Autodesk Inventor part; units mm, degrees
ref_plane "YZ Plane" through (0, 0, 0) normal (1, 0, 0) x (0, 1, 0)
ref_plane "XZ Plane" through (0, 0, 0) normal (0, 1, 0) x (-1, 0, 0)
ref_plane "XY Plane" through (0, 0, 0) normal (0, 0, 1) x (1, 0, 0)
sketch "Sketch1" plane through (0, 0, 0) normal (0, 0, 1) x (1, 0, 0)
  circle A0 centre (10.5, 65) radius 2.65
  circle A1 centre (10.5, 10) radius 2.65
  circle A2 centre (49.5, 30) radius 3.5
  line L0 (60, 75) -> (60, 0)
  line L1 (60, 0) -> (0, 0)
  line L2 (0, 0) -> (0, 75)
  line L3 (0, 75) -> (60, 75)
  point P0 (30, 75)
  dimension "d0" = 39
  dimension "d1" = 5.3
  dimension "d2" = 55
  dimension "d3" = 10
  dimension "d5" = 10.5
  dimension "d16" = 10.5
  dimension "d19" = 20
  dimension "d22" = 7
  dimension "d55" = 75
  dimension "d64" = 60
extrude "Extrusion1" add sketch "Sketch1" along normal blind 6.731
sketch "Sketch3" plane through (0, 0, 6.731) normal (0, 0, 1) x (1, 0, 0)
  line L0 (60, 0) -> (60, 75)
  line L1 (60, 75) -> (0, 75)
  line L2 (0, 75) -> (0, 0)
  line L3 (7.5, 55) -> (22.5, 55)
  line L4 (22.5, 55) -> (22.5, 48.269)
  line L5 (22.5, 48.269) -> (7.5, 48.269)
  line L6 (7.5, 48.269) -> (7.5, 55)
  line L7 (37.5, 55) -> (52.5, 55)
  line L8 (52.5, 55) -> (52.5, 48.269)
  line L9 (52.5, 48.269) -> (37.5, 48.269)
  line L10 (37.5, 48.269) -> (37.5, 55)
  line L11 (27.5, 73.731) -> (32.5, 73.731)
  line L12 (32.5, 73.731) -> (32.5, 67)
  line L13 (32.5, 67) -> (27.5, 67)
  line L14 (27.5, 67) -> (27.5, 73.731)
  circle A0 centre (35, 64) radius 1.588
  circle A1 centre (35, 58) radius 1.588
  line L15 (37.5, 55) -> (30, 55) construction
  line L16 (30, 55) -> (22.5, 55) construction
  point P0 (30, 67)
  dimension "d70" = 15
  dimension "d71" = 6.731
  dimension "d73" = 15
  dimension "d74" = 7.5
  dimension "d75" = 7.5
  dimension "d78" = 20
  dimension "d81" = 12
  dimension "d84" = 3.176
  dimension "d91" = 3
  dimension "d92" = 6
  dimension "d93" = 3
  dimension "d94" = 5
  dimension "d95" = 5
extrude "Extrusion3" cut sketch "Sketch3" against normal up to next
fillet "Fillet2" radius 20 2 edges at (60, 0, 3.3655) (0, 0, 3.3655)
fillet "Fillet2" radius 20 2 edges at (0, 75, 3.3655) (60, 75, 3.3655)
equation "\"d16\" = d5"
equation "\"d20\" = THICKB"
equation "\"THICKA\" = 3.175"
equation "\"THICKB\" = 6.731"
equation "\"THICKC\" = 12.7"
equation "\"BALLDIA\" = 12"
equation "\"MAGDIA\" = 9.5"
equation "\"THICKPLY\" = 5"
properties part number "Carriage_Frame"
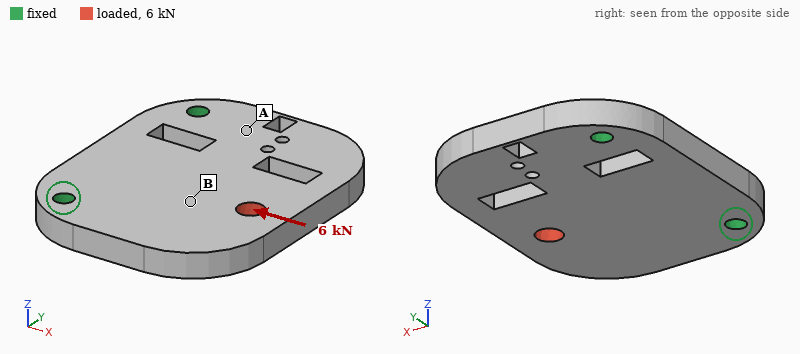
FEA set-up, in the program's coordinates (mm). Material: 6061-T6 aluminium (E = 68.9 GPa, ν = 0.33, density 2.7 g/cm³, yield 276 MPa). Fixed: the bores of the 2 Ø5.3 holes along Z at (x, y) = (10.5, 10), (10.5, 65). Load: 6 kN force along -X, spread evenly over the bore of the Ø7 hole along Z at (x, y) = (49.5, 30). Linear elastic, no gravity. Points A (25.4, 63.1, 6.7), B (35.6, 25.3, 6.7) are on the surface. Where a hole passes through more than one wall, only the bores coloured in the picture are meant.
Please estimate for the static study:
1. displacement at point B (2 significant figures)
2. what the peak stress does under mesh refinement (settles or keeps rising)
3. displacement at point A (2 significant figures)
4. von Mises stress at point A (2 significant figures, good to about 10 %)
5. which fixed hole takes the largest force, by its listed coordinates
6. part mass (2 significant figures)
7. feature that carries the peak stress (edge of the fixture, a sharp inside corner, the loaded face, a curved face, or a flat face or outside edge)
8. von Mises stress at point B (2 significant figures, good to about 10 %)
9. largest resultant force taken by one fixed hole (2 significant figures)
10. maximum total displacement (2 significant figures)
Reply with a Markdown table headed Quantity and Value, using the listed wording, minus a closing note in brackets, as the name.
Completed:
| Quantity | Value |
|---|---|
| displacement at point B | 15 µm |
| what the peak stress does under mesh refinement | keeps rising |
| displacement at point A | 4.3 µm |
| von Mises stress at point A | 11 MPa |
| which fixed hole takes the largest force, by its listed coordinates | (10.5, 10) |
| part mass | 69 g |
| feature that carries the peak stress | edge of the fixture |
| von Mises stress at point B | 28 MPa |
| largest resultant force taken by one fixed hole | 3.9 kN |
| maximum total displacement | 27 µm |
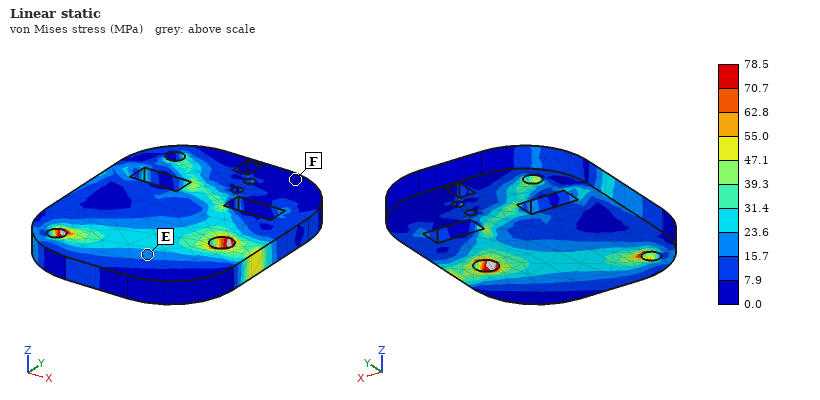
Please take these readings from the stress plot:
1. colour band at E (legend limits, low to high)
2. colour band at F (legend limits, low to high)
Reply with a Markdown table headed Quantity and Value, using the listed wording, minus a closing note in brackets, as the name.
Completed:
| Quantity | Value |
|---|---|
| colour band at E | 15.7 to 23.6 MPa |
| colour band at F | 0.0 to 7.9 MPa |
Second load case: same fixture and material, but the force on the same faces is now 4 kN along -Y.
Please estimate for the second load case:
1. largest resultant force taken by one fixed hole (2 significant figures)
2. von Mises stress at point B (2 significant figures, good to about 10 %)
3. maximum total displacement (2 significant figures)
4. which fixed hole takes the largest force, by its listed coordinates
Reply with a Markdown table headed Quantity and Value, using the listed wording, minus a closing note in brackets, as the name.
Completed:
| Quantity | Value |
|---|---|
| largest resultant force taken by one fixed hole | 3.5 kN |
| von Mises stress at point B | 20 MPa |
| maximum total displacement | 36 µm |
| which fixed hole takes the largest force, by its listed coordinates | (10.5, 10) |
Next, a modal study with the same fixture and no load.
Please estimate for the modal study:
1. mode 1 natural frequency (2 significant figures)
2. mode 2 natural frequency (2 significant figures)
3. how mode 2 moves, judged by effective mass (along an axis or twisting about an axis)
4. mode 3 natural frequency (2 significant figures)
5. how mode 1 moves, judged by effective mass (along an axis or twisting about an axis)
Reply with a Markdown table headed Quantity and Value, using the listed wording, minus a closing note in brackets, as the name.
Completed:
| Quantity | Value |
|---|---|
| mode 1 natural frequency | 2000 Hz |
| mode 2 natural frequency | 4400 Hz |
| how mode 2 moves, judged by effective mass | twisting about X |
| mode 3 natural frequency | 8400 Hz |
| how mode 1 moves, judged by effective mass | along Z |
